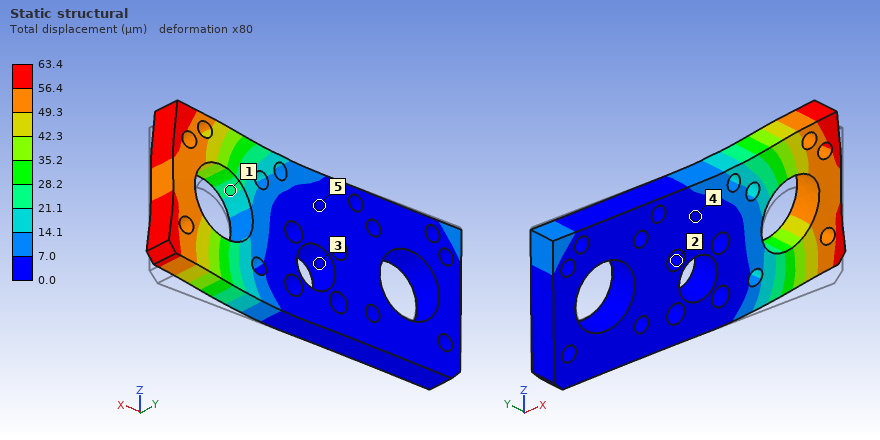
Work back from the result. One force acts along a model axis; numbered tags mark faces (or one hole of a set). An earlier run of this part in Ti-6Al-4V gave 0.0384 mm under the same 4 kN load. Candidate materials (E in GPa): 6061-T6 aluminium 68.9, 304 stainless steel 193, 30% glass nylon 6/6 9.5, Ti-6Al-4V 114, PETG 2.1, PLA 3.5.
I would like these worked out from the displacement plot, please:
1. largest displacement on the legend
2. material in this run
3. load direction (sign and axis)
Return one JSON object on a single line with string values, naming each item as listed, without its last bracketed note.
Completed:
{"largest displacement on the legend": "63.4 µm", "material in this run": "6061-T6 aluminium", "load direction": "+Z"}
